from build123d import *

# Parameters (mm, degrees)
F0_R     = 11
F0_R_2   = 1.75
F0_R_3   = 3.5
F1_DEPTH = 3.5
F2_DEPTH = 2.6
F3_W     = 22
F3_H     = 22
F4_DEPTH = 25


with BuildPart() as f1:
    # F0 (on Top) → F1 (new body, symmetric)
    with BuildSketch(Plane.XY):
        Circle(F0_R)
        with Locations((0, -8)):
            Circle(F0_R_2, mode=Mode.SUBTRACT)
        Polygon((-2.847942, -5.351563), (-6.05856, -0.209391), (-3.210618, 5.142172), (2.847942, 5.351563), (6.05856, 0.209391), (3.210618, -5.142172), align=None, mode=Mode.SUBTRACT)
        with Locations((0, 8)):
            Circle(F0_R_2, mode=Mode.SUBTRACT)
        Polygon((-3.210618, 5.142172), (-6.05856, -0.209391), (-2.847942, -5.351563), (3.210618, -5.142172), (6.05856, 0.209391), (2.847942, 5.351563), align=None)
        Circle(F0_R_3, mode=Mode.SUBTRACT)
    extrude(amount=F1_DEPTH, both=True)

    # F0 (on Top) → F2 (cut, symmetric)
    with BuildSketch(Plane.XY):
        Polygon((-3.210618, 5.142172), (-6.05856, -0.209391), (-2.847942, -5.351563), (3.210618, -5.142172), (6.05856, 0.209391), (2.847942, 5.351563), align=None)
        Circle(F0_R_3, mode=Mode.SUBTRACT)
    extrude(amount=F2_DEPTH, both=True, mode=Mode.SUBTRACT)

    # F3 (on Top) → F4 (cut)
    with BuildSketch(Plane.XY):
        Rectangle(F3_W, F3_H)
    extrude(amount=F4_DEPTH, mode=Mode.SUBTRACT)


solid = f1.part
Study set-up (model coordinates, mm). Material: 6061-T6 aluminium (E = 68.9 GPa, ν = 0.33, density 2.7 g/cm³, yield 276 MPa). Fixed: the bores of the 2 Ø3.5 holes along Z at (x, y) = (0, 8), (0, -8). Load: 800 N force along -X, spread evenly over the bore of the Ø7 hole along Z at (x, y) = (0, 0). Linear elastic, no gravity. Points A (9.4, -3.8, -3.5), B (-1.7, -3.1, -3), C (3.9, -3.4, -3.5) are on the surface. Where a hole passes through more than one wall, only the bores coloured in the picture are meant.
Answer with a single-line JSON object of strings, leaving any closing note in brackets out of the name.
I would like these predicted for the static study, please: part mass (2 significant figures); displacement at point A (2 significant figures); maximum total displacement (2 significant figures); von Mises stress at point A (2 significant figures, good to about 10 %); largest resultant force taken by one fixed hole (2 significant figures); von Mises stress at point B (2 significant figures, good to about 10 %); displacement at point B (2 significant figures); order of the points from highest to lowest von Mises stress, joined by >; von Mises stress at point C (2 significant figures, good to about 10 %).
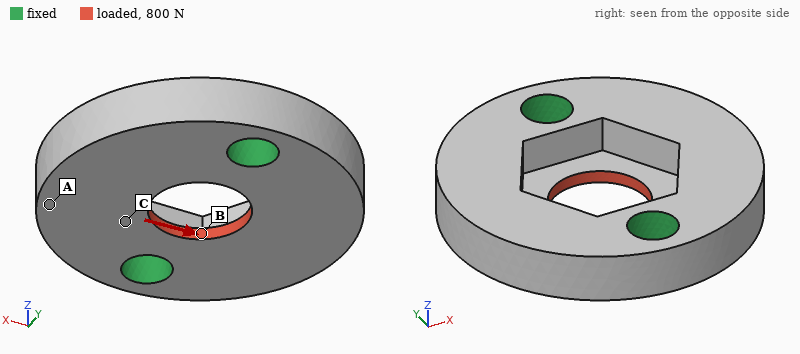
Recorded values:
{"part mass": "2.6 g", "displacement at point A": "5.5 µm", "maximum total displacement": "7.1 µm", "von Mises stress at point A": "11 MPa", "largest resultant force taken by one fixed hole": "400 N", "von Mises stress at point B": "68 MPa", "displacement at point B": "4.2 µm", "order of the points from highest to lowest von Mises stress, joined by >": "B > C > A", "von Mises stress at point C": "34 MPa"}
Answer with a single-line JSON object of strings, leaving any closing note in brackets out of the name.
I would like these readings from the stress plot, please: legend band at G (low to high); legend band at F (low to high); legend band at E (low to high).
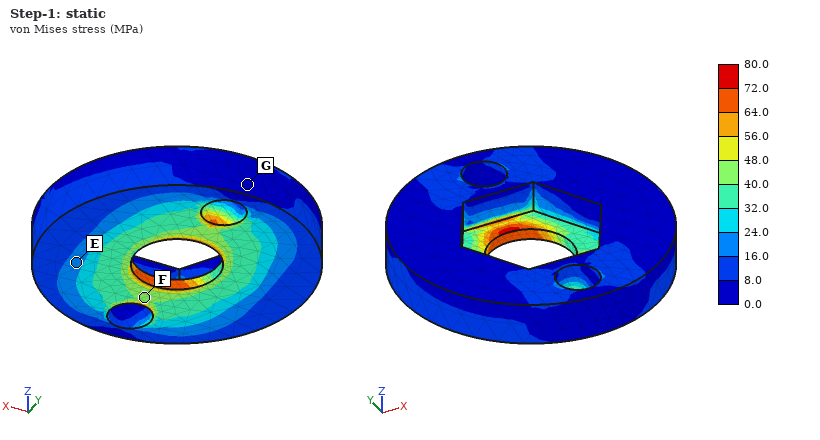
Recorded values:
{"legend band at G": "0.0 to 8.0 MPa", "legend band at F": "40.0 to 48.0 MPa", "legend band at E": "16.0 to 24.0 MPa"}
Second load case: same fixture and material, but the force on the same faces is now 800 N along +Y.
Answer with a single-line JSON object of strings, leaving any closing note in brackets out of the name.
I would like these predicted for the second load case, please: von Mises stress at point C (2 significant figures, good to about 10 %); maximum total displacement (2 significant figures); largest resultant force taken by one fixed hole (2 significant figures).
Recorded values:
{"von Mises stress at point C": "27 MPa", "maximum total displacement": "4.0 µm", "largest resultant force taken by one fixed hole": "400 N"}
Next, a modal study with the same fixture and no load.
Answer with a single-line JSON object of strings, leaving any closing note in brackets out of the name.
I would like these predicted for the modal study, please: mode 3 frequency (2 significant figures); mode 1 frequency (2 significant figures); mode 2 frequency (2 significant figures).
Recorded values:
{"mode 3 frequency": "56 kHz", "mode 1 frequency": "24 kHz", "mode 2 frequency": "25 kHz"}
